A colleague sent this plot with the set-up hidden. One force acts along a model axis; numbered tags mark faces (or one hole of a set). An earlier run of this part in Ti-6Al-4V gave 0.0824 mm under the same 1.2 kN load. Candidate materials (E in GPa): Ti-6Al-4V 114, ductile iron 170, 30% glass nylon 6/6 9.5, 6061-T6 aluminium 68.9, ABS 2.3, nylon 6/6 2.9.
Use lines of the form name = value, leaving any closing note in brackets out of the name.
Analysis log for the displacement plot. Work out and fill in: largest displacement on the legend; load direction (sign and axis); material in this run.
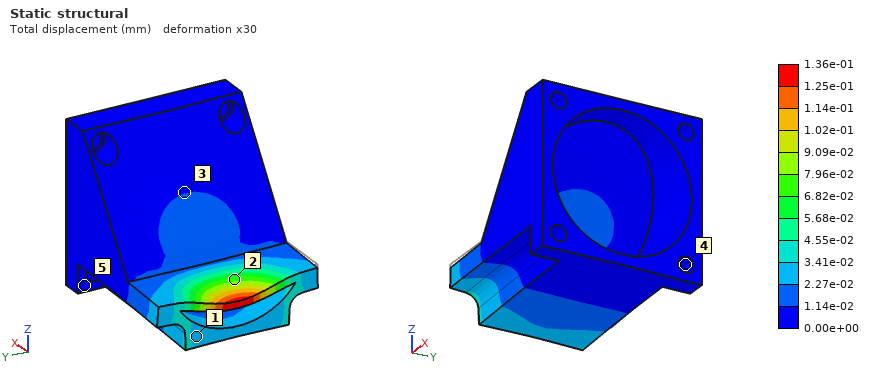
largest displacement on the legend = 1.36e-01 mm
load direction = -Z
material in this run = 6061-T6 aluminium
